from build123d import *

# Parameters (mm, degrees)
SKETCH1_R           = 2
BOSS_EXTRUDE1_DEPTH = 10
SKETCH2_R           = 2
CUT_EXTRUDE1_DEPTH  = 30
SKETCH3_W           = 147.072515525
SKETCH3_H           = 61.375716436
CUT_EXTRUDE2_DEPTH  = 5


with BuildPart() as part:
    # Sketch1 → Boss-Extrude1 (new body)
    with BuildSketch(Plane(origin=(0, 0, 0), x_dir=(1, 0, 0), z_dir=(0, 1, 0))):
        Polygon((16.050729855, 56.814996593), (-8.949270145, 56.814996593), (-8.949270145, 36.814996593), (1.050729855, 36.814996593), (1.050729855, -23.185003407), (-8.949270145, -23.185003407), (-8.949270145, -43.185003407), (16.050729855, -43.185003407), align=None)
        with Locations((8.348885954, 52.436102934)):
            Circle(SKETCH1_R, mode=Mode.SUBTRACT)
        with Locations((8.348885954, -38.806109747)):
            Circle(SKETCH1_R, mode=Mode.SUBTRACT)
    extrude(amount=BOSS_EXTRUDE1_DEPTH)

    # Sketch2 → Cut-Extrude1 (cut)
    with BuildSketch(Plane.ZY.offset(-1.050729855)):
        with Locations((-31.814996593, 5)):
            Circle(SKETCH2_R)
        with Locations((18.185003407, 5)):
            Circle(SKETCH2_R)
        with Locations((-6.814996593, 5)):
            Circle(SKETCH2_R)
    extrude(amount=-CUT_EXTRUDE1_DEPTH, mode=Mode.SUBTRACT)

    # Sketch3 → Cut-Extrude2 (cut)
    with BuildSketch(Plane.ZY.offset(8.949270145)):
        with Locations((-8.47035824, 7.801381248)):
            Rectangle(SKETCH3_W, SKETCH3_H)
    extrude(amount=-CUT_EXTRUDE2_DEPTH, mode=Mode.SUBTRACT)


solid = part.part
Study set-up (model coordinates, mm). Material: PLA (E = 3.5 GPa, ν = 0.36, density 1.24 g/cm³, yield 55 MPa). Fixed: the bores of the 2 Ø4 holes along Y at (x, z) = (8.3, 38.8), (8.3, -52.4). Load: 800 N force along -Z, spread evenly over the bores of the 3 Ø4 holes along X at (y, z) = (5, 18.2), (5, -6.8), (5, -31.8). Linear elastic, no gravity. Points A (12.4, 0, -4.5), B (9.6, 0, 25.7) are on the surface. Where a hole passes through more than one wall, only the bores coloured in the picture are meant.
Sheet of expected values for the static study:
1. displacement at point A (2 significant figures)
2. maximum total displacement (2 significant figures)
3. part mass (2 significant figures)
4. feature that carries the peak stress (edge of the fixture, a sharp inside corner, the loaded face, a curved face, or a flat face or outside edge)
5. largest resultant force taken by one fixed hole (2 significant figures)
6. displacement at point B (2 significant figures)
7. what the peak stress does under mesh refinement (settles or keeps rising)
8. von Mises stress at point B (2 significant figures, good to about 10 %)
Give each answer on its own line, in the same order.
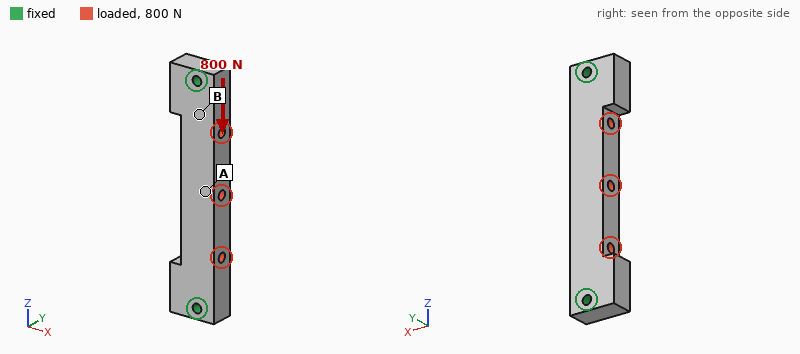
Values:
25 µm
26 µm
20 g
edge of the fixture
400 N
12 µm
keeps rising
3.0 MPa
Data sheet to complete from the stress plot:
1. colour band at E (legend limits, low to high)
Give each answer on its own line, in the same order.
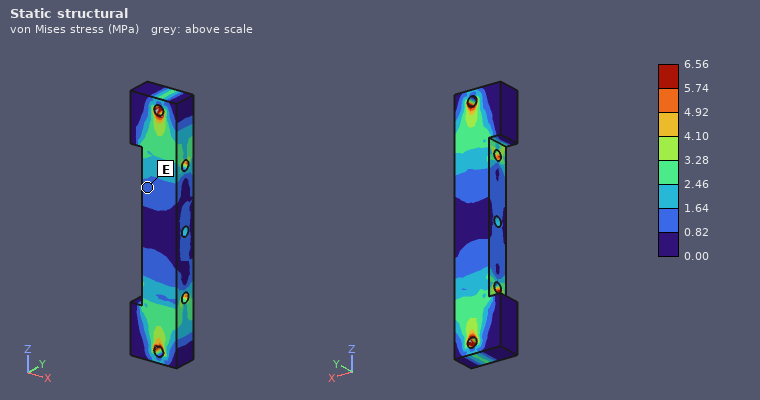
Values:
0.82 to 1.64 MPa
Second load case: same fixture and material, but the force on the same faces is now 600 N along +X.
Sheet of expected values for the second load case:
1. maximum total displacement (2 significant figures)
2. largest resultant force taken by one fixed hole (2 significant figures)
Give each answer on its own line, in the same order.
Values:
0.33 mm
300 N
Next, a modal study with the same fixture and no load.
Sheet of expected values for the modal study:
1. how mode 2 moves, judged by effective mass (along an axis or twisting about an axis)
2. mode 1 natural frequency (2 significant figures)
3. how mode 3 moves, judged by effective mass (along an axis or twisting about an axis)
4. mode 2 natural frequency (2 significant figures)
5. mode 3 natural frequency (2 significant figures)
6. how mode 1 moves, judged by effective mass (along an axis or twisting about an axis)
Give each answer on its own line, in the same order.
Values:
along X
1900 Hz
twisting about X
2100 Hz
4800 Hz
along Y
